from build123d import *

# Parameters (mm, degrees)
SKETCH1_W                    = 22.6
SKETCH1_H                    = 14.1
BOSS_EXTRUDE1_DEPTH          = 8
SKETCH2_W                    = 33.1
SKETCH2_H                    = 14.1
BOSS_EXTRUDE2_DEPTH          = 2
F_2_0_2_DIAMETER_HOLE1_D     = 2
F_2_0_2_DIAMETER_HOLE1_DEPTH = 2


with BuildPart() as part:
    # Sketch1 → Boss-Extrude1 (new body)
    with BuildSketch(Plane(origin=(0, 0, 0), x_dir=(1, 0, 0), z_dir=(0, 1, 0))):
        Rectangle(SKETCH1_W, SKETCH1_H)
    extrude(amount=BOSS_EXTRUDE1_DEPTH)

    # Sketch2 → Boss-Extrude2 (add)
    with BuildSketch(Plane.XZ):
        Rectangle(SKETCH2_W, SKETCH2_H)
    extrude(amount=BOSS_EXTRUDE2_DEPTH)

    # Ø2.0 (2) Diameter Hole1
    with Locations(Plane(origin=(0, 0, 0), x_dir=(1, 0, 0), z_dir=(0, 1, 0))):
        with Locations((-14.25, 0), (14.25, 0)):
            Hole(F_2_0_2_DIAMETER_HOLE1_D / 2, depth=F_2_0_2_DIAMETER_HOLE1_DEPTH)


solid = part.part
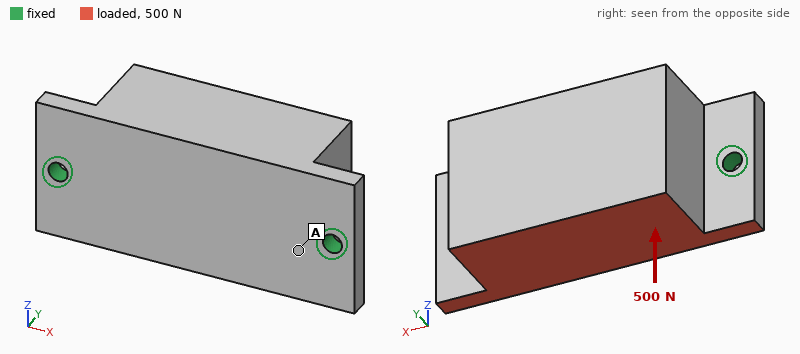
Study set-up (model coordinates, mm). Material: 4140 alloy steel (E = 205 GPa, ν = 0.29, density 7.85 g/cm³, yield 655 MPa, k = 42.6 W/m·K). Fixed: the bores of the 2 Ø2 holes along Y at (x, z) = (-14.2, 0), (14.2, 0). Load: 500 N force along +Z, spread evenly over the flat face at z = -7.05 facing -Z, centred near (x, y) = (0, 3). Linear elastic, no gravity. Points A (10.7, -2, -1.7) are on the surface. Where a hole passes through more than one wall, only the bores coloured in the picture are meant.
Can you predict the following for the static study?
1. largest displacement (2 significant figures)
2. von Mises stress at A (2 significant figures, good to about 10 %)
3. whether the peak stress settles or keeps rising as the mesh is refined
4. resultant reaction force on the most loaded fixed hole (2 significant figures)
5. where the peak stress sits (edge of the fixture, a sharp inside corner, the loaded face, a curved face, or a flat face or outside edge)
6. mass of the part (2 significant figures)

15 µm
25 MPa
keeps rising
250 N
edge of the fixture
27 g
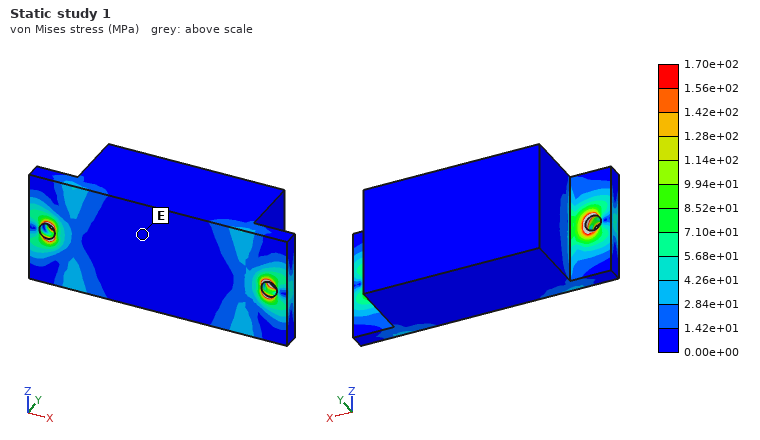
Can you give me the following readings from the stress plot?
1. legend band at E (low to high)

0.00e+00 to 1.42e+01 MPa
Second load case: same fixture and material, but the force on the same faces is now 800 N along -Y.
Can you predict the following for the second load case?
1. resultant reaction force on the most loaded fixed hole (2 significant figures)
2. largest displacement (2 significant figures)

450 N
45 µm
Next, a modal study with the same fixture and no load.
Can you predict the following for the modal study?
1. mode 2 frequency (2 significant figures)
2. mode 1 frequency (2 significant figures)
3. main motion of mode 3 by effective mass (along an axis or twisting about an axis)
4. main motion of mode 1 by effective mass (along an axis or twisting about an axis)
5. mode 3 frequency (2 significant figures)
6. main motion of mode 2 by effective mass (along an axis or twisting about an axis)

15 kHz
5900 Hz
along X
along Z
23 kHz
along Y
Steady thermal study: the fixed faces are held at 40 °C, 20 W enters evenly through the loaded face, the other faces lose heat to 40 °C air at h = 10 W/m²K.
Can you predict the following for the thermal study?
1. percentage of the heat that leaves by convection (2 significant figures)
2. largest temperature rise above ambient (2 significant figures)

3.4 %
68 K
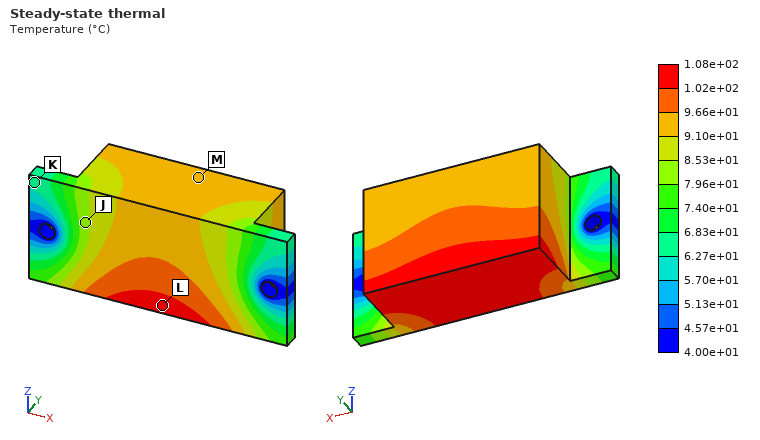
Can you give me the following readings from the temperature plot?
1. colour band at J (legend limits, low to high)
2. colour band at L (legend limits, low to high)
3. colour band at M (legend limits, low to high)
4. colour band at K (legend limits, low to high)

7.96e+01 to 8.53e+01 °C
1.02e+02 to 1.08e+02 °C
9.10e+01 to 9.66e+01 °C
6.27e+01 to 6.83e+01 °C
